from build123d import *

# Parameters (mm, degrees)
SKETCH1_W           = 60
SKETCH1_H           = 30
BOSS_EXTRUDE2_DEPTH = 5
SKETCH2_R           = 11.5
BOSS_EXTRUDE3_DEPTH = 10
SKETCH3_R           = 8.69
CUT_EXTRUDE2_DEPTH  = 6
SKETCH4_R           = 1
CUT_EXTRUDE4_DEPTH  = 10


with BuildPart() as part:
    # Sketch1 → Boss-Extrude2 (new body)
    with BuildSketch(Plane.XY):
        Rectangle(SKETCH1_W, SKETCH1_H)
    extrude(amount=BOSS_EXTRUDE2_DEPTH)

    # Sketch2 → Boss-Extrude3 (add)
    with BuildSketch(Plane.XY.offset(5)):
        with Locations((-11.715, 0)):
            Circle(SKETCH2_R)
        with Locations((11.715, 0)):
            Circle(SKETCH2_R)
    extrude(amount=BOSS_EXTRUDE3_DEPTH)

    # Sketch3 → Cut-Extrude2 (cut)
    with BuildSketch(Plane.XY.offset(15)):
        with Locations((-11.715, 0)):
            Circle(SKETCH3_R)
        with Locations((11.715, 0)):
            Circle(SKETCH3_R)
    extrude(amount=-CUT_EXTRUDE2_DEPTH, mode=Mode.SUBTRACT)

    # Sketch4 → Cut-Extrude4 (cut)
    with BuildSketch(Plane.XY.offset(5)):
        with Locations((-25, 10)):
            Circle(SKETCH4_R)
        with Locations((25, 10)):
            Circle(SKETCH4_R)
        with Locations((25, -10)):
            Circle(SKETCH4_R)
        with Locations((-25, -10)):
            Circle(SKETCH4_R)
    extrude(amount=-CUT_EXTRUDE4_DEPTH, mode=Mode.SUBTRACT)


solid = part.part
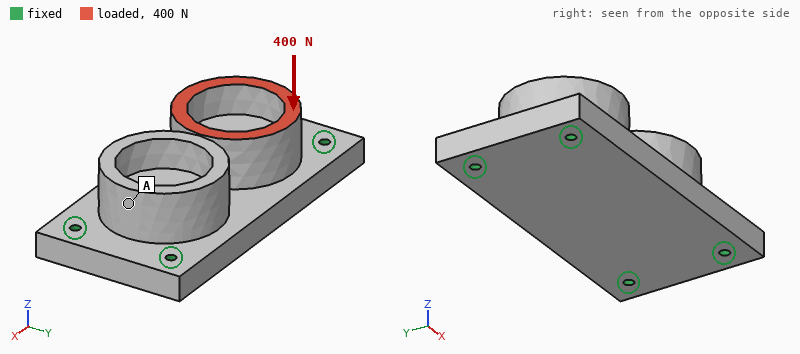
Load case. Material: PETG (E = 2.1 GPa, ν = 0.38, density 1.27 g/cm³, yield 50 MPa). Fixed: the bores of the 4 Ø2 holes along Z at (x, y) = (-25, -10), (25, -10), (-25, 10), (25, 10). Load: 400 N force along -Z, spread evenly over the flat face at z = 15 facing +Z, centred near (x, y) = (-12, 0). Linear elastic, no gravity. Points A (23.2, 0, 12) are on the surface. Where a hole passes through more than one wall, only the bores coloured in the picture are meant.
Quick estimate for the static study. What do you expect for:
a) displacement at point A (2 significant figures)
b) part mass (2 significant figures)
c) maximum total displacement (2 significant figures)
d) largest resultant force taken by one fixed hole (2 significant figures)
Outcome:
0.087 mm
18 g
0.27 mm
160 N
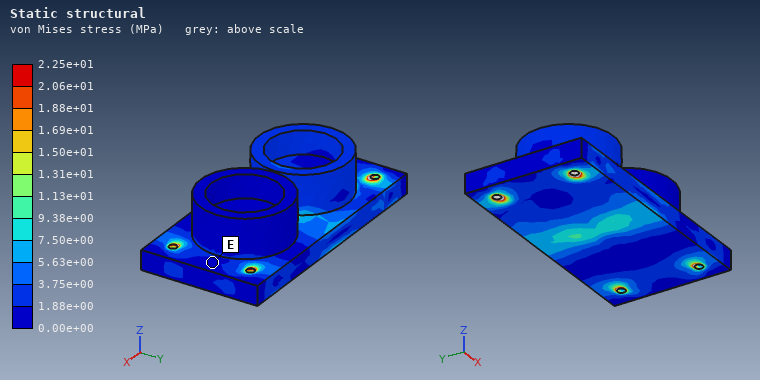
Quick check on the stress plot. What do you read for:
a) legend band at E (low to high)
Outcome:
0.00e+00 to 1.88e+00 MPa
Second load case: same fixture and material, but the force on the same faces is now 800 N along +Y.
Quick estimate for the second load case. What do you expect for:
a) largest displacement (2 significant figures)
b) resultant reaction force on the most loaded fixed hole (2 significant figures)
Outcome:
0.55 mm
510 N
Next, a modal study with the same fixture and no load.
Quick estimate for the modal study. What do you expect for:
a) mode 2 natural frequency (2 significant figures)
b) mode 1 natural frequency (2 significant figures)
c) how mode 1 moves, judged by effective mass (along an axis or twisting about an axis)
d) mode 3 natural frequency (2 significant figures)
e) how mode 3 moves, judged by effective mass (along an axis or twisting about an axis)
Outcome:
3600 Hz
1900 Hz
along Z
4900 Hz
along Y
